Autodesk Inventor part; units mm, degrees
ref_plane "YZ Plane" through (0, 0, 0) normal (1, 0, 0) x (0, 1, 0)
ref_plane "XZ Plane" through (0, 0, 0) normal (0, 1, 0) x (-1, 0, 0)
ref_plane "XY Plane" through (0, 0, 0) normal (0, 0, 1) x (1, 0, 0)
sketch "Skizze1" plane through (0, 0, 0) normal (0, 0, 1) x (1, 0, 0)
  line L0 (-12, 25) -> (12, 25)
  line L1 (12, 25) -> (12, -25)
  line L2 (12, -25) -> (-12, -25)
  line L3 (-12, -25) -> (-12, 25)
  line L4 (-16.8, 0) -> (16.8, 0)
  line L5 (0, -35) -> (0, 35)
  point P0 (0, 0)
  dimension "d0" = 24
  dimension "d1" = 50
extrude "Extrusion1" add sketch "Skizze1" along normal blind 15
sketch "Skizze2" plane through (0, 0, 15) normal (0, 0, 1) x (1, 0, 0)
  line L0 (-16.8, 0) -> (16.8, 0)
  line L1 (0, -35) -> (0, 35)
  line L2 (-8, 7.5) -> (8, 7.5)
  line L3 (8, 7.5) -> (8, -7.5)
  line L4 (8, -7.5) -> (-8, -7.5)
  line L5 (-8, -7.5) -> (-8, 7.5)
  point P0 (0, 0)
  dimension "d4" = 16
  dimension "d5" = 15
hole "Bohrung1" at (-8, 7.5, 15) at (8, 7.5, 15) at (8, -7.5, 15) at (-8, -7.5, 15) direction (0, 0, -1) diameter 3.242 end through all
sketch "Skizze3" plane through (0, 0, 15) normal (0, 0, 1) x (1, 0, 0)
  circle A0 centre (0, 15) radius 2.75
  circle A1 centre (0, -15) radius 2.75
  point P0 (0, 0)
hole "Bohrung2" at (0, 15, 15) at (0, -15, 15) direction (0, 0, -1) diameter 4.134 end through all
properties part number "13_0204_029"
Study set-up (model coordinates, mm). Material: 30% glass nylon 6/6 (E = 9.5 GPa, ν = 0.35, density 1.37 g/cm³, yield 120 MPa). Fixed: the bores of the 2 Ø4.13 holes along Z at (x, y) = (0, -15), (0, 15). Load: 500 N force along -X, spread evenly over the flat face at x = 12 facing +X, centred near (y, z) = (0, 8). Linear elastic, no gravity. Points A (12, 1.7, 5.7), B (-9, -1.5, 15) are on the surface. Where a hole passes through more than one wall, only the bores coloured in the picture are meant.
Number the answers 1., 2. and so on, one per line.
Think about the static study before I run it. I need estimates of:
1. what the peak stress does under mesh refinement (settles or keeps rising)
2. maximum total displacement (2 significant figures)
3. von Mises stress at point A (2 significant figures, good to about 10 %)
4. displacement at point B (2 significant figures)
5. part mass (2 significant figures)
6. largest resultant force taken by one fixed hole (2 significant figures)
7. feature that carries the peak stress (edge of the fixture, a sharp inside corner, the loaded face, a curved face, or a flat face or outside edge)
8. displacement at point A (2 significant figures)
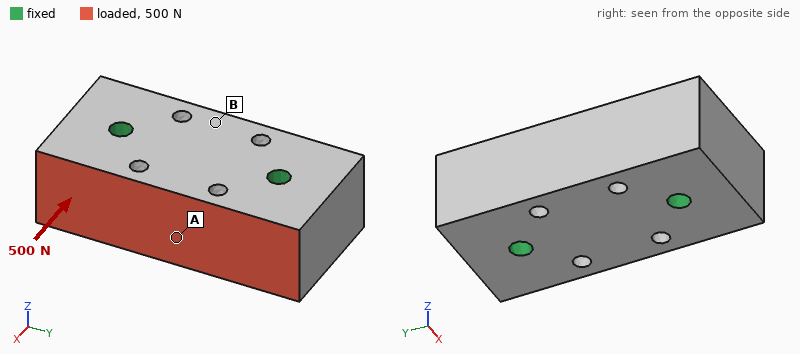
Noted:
1. keeps rising
2. 2.0 µm
3. 0.61 MPa
4. 1.2 µm
5. 23 g
6. 250 N
7. edge of the fixture
8. 1.9 µm
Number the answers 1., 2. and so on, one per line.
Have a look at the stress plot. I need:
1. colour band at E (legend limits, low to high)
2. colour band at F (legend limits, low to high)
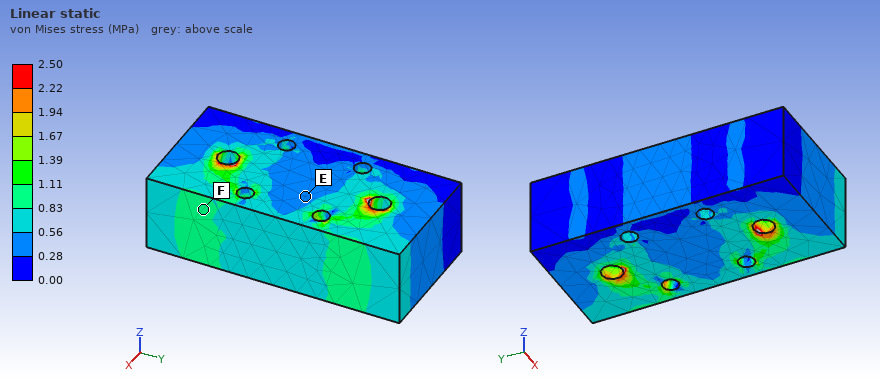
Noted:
1. 0.28 to 0.56 MPa
2. 0.83 to 1.11 MPa
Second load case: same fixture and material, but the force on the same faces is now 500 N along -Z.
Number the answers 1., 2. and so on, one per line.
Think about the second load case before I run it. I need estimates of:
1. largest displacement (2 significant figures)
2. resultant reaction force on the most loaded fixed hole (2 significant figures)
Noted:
1. 11 µm
2. 250 N
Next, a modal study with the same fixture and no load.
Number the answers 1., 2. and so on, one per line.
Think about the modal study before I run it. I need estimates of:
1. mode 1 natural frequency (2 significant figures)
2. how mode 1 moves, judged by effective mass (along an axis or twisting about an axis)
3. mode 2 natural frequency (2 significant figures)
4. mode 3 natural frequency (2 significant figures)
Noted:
1. 17 kHz
2. twisting about Y
3. 18 kHz
4. 18 kHz
